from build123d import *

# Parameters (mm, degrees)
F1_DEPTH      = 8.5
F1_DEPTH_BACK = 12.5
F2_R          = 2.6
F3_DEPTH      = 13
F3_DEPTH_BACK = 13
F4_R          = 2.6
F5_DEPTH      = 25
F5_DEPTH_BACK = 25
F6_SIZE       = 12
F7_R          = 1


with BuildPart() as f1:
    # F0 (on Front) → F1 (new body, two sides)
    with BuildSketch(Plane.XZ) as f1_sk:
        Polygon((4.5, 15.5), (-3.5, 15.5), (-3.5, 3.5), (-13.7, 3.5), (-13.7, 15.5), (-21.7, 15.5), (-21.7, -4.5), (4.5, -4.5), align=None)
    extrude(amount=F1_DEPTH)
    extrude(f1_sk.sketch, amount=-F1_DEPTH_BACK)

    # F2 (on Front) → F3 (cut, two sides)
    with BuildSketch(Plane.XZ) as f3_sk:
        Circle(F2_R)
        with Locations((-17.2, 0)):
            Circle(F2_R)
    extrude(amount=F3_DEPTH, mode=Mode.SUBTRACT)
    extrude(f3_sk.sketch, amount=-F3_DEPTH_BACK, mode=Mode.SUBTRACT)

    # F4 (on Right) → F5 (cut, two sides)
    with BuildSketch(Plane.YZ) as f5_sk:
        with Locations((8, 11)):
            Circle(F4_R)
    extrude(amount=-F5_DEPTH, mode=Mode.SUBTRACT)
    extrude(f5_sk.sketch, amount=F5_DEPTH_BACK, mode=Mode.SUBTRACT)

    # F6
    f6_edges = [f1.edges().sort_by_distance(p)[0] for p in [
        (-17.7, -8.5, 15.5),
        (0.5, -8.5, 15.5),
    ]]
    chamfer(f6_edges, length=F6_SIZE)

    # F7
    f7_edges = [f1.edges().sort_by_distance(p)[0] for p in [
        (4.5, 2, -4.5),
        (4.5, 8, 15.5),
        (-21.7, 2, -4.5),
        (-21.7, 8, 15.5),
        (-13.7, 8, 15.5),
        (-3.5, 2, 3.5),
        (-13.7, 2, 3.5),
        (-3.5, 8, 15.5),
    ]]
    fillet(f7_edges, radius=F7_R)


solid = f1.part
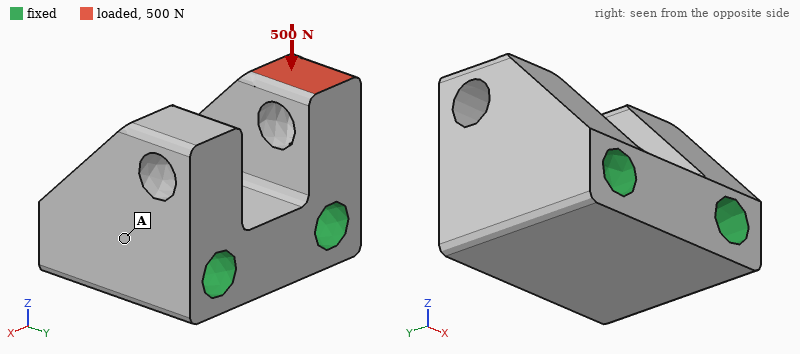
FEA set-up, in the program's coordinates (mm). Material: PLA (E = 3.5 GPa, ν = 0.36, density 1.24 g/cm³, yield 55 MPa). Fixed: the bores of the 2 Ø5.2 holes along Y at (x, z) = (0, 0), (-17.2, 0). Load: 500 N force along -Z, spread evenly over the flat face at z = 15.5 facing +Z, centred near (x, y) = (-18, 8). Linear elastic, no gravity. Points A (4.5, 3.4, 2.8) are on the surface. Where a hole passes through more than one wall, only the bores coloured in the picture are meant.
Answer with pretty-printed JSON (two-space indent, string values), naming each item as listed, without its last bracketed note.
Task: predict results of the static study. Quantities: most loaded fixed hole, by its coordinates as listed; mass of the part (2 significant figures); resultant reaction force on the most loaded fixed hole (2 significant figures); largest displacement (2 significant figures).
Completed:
{
  "most loaded fixed hole, by its coordinates as listed": "(-17.2, 0)",
  "mass of the part": "7.5 g",
  "resultant reaction force on the most loaded fixed hole": "490 N",
  "largest displacement": "75 µm"
}
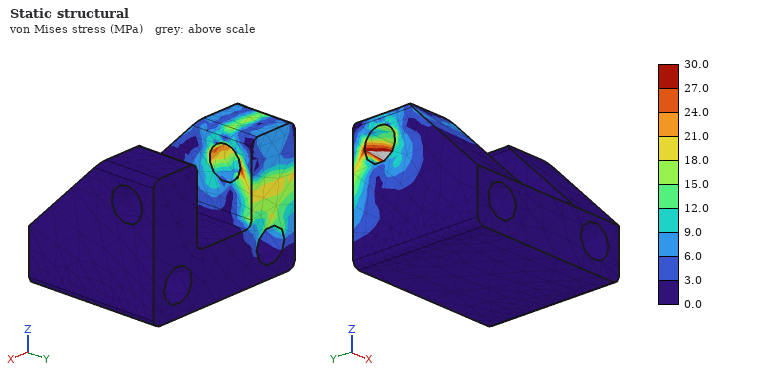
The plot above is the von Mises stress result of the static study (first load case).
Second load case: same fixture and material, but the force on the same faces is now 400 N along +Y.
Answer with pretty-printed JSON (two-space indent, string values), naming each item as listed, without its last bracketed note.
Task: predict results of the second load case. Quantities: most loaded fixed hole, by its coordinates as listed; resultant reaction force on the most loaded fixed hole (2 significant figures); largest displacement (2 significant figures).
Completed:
{
  "most loaded fixed hole, by its coordinates as listed": "(-17.2, 0)",
  "resultant reaction force on the most loaded fixed hole": "400 N",
  "largest displacement": "0.13 mm"
}
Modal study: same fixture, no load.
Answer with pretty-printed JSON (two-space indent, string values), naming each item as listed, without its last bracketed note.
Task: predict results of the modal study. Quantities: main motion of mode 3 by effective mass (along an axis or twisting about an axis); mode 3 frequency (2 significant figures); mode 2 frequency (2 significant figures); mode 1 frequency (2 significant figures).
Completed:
{
  "main motion of mode 3 by effective mass": "along Y",
  "mode 3 frequency": "17 kHz",
  "mode 2 frequency": "11 kHz",
  "mode 1 frequency": "11 kHz"
}
